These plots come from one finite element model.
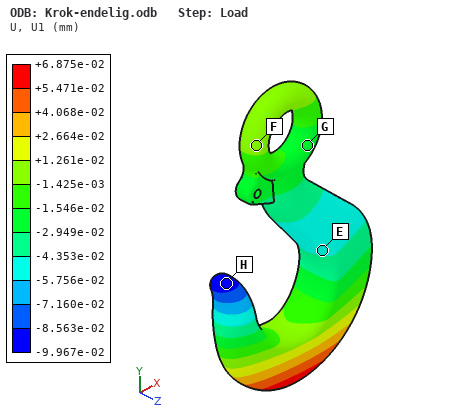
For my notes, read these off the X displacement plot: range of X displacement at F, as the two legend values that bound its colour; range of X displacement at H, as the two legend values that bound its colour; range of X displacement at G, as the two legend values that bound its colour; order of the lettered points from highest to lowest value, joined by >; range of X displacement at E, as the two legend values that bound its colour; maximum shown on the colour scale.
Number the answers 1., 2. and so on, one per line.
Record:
1. -1.425e-03 to +1.261e-02 mm
2. -9.967e-02 to -8.563e-02 mm
3. -2.949e-02 to -1.546e-02 mm
4. F > G > E > H
5. -5.756e-02 to -4.353e-02 mm
6. +6.875e-02 mm
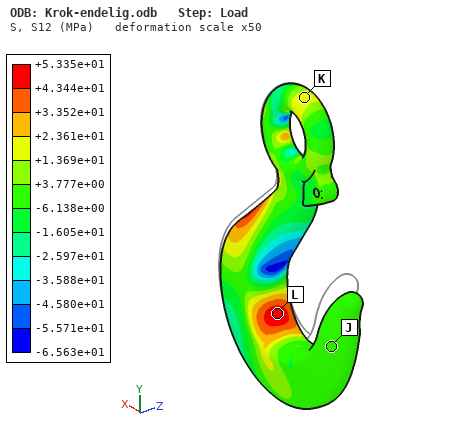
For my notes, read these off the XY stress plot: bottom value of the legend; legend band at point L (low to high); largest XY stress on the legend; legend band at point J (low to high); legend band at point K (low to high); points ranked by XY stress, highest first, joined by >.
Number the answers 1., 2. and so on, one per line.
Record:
1. -6.563e+01 MPa
2. +4.344e+01 to +5.335e+01 MPa
3. +5.335e+01 MPa
4. -6.138e+00 to +3.777e+00 MPa
5. +1.369e+01 to +2.361e+01 MPa
6. L > K > J
